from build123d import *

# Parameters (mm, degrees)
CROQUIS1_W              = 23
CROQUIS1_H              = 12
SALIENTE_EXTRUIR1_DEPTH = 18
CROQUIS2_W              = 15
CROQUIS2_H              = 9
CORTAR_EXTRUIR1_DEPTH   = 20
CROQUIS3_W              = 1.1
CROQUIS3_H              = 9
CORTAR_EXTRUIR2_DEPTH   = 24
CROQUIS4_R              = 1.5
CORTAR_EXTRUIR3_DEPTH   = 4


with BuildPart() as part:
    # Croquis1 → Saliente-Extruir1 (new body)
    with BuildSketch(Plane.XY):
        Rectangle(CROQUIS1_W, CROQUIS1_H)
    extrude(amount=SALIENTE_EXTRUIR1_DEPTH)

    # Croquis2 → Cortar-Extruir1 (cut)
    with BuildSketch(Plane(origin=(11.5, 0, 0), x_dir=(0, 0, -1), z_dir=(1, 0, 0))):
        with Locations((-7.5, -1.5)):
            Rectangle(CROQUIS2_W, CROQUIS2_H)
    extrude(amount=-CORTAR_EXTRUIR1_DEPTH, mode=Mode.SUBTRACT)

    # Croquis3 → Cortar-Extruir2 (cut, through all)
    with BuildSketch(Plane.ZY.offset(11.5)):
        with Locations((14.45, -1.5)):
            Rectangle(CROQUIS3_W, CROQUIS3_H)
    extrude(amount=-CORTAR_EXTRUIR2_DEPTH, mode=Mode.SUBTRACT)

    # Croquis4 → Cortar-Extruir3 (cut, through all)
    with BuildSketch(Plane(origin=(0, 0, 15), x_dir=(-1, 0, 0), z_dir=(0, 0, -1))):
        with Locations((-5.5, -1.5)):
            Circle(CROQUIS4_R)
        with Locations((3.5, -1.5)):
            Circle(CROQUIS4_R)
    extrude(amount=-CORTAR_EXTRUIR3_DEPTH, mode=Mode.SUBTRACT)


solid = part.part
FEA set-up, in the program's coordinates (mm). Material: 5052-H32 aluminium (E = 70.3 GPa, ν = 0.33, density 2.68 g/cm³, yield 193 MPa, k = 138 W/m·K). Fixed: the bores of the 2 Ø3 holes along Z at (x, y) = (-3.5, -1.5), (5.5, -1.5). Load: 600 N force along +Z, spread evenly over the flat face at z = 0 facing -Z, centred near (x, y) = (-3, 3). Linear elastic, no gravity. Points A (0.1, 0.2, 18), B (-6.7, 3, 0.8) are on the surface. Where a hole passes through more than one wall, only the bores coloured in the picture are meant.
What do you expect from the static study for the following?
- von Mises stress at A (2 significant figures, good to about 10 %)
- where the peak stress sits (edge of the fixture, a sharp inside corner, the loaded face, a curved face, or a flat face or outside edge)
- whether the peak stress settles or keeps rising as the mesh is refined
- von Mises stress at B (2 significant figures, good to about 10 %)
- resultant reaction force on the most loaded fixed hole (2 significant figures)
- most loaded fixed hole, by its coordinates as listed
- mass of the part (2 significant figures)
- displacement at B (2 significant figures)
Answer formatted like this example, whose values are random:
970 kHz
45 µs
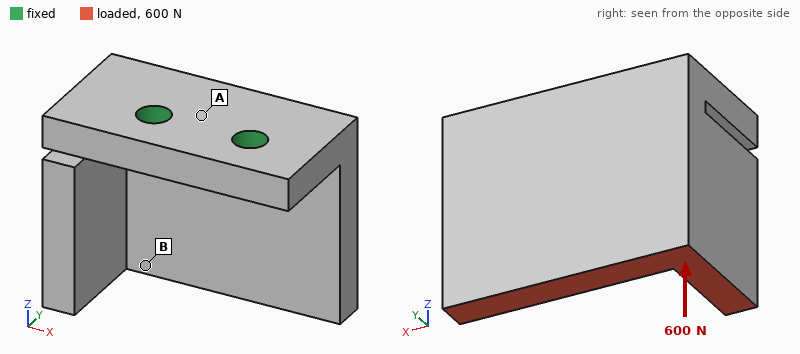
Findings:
30 MPa
edge of the fixture
keeps rising
13 MPa
470 N
(-3.5, -1.5)
5.9 g
18 µm
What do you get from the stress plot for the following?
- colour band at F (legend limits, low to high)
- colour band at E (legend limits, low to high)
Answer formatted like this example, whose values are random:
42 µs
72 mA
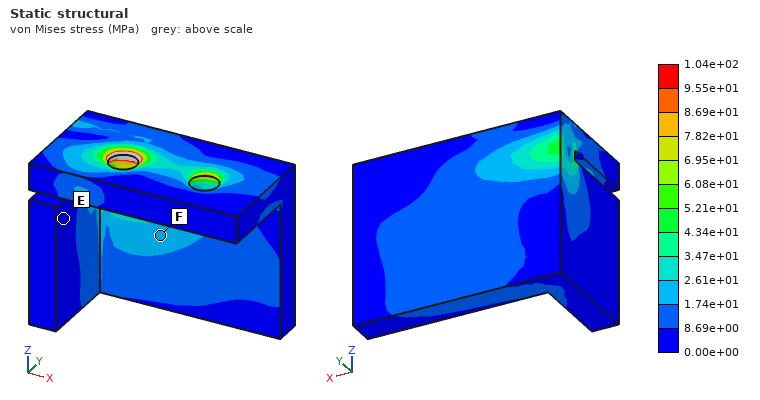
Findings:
1.74e+01 to 2.61e+01 MPa
0.00e+00 to 8.69e+00 MPa
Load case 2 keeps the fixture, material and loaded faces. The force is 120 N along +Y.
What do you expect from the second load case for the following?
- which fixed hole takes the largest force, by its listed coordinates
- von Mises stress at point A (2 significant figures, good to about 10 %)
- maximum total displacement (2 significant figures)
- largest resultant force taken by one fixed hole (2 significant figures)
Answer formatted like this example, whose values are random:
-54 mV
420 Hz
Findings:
(-3.5, -1.5)
39 MPa
0.10 mm
100 N
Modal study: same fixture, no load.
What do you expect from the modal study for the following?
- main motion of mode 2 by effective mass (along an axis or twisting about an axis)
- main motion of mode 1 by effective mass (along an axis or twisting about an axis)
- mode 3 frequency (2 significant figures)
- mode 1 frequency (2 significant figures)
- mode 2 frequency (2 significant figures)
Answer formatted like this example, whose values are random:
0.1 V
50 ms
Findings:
along X
along Y
12 kHz
5000 Hz
8500 Hz
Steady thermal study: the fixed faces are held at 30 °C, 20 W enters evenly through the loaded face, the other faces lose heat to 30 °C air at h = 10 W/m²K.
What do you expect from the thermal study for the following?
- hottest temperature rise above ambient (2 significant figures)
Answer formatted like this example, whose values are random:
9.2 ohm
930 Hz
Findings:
45 K
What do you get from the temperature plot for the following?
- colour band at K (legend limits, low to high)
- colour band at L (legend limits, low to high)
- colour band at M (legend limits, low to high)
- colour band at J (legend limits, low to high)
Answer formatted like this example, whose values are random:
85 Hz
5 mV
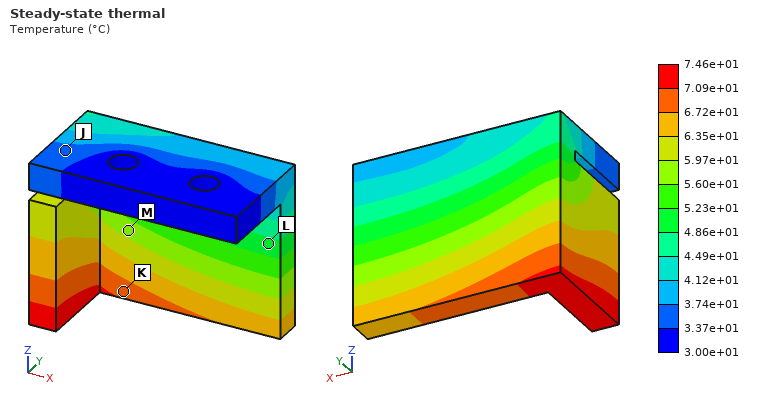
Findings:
6.72e+01 to 7.09e+01 °C
4.86e+01 to 5.23e+01 °C
5.60e+01 to 5.97e+01 °C
3.37e+01 to 3.74e+01 °C
